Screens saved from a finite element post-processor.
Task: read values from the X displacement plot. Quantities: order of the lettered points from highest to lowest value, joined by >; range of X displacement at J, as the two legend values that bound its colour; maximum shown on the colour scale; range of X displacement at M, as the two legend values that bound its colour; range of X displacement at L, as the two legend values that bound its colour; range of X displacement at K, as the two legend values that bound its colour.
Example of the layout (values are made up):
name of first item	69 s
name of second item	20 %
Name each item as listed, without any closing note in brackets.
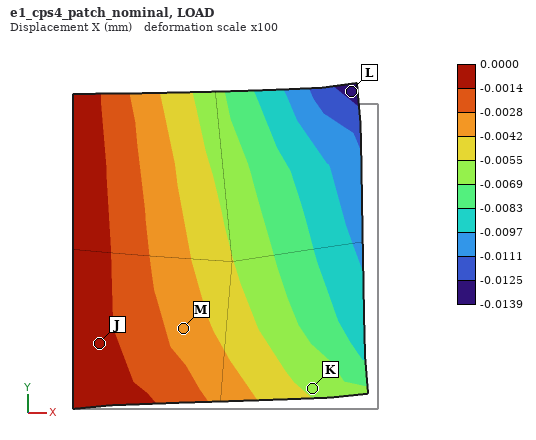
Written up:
order of the lettered points from highest to lowest value, joined by >	J > M > K > L
range of X displacement at J, as the two legend values that bound its colour	-0.0014 to 0.0000 mm
maximum shown on the colour scale	0.0000 mm
range of X displacement at M, as the two legend values that bound its colour	-0.0042 to -0.0028 mm
range of X displacement at L, as the two legend values that bound its colour	-0.0139 to -0.0125 mm
range of X displacement at K, as the two legend values that bound its colour	-0.0069 to -0.0055 mm
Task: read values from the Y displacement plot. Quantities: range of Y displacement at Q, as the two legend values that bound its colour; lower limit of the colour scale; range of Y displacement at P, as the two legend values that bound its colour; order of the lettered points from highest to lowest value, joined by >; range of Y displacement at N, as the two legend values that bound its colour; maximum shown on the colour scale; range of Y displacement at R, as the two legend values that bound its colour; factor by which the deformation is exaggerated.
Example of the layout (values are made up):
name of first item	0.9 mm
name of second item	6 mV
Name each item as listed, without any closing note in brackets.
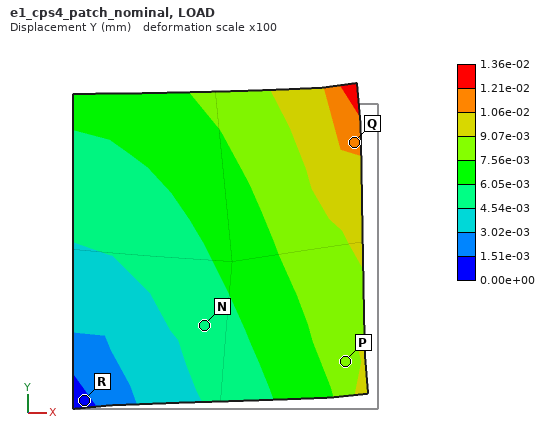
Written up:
range of Y displacement at Q, as the two legend values that bound its colour	1.06e-02 to 1.21e-02 mm
lower limit of the colour scale	0.00e+00 mm
range of Y displacement at P, as the two legend values that bound its colour	7.56e-03 to 9.07e-03 mm
order of the lettered points from highest to lowest value, joined by >	Q > P > N > R
range of Y displacement at N, as the two legend values that bound its colour	4.54e-03 to 6.05e-03 mm
maximum shown on the colour scale	1.36e-02 mm
range of Y displacement at R, as the two legend values that bound its colour	0.00e+00 to 1.51e-03 mm
factor by which the deformation is exaggerated	100
